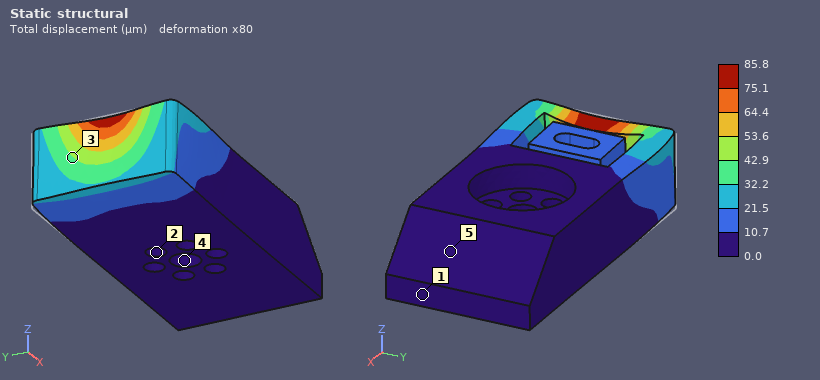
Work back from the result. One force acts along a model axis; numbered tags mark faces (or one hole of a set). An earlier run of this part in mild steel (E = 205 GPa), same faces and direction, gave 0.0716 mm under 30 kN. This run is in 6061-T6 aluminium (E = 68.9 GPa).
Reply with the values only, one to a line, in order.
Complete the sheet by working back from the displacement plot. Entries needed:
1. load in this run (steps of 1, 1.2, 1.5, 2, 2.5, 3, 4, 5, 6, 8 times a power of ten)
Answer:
12 kN
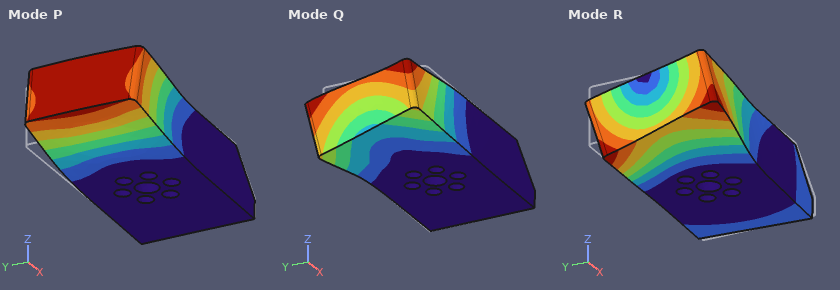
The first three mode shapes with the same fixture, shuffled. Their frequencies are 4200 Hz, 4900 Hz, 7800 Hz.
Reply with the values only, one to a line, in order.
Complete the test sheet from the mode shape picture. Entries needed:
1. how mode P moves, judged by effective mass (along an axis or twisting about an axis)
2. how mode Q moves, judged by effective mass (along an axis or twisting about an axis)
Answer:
along Z
along Y
